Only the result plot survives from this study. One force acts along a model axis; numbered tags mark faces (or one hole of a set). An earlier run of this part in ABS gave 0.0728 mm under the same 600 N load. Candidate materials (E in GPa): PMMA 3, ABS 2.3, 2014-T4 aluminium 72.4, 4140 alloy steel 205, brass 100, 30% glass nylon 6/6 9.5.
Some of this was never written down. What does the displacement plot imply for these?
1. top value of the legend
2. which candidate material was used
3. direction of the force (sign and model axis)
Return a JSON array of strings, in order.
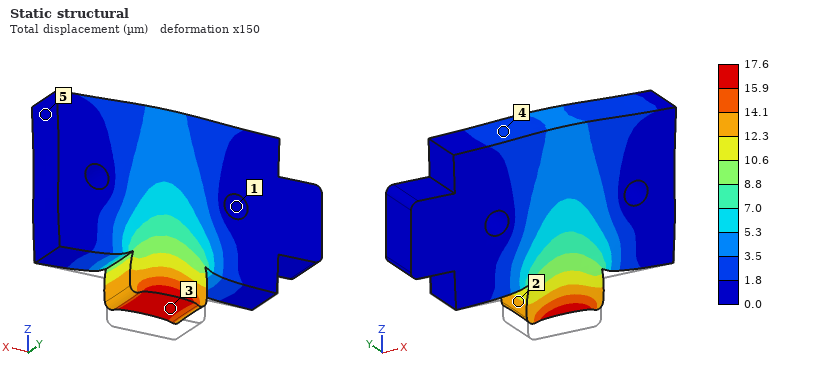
["17.6 µm", "30% glass nylon 6/6", "+Z"]
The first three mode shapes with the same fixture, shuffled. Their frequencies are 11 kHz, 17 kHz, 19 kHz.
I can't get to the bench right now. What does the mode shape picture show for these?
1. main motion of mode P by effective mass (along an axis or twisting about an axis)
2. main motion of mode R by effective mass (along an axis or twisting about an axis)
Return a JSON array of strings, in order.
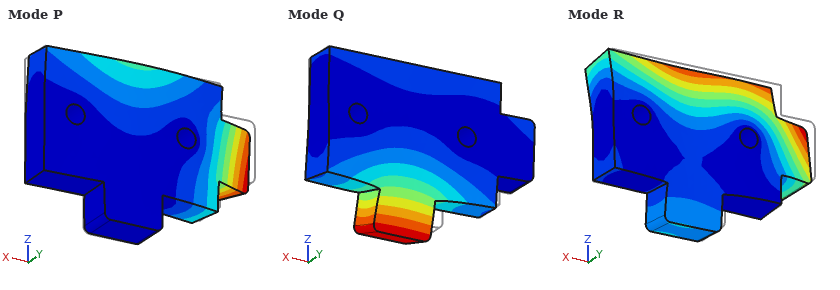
["twisting about Z", "along Y"]
